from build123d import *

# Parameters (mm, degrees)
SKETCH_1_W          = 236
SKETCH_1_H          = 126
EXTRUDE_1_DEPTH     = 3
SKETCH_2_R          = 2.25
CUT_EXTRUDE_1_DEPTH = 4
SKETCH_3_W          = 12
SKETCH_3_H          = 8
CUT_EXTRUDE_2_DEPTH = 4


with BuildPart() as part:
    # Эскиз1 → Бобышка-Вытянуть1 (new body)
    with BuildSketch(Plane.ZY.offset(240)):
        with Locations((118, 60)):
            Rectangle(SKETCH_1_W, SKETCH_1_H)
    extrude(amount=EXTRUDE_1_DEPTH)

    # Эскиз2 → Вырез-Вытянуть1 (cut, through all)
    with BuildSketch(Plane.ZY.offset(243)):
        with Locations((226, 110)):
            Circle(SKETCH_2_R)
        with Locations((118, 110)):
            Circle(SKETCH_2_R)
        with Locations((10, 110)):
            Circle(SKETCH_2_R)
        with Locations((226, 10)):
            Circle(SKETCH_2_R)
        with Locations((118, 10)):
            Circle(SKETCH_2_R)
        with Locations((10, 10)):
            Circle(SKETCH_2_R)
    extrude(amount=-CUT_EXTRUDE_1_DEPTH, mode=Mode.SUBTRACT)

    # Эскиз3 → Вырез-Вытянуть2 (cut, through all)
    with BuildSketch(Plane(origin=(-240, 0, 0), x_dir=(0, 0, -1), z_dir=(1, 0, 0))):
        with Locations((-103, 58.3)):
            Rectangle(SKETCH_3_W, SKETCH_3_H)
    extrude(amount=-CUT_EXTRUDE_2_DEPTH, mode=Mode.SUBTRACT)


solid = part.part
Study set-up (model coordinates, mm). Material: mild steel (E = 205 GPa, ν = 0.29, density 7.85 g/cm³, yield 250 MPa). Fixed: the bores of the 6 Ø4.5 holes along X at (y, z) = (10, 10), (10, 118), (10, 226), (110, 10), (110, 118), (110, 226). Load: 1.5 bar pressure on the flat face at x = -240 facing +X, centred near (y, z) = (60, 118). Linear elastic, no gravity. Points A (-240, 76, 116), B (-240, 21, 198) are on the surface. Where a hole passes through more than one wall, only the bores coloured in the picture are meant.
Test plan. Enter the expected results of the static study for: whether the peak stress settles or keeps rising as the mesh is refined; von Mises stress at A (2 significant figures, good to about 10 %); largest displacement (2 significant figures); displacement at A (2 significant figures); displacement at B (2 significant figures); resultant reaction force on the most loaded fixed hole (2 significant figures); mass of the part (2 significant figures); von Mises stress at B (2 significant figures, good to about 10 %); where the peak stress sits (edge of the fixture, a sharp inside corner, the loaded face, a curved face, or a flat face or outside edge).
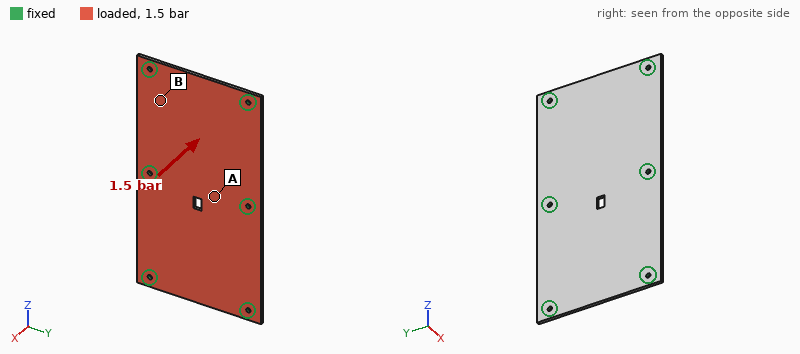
keeps rising
69 MPa
0.25 mm
0.15 mm
0.13 mm
1.1 kN
700 g
32 MPa
edge of the fixture
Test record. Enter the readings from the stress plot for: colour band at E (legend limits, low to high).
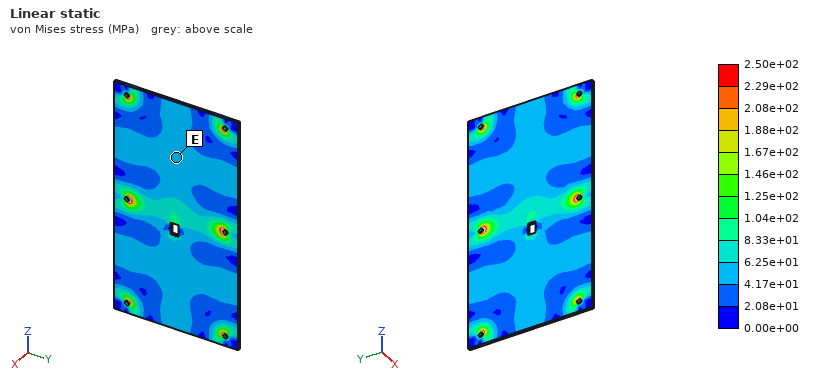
4.17e+01 to 6.25e+01 MPa
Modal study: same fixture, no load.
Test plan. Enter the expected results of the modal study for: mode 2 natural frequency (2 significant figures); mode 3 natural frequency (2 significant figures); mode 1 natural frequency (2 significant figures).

970 Hz
1500 Hz
960 Hz
